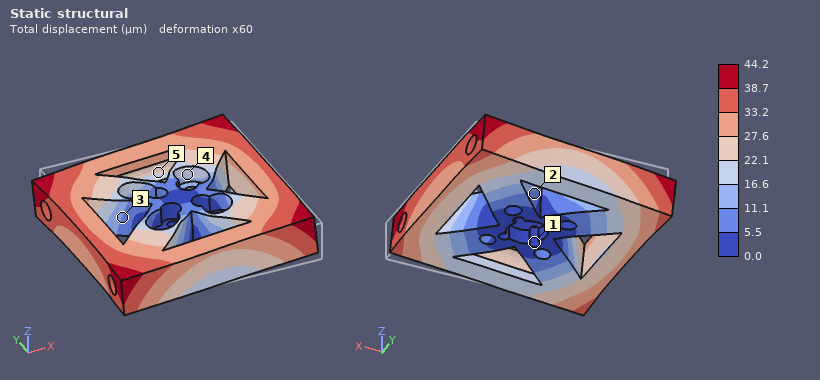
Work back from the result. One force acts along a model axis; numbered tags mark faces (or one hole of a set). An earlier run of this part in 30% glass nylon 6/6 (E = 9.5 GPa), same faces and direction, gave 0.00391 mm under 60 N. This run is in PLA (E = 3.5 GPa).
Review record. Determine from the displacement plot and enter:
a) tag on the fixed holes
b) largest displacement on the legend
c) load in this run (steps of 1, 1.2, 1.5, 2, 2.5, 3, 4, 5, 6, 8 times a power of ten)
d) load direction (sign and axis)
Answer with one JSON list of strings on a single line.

["1", "44.2 µm", "250 N", "-X"]
